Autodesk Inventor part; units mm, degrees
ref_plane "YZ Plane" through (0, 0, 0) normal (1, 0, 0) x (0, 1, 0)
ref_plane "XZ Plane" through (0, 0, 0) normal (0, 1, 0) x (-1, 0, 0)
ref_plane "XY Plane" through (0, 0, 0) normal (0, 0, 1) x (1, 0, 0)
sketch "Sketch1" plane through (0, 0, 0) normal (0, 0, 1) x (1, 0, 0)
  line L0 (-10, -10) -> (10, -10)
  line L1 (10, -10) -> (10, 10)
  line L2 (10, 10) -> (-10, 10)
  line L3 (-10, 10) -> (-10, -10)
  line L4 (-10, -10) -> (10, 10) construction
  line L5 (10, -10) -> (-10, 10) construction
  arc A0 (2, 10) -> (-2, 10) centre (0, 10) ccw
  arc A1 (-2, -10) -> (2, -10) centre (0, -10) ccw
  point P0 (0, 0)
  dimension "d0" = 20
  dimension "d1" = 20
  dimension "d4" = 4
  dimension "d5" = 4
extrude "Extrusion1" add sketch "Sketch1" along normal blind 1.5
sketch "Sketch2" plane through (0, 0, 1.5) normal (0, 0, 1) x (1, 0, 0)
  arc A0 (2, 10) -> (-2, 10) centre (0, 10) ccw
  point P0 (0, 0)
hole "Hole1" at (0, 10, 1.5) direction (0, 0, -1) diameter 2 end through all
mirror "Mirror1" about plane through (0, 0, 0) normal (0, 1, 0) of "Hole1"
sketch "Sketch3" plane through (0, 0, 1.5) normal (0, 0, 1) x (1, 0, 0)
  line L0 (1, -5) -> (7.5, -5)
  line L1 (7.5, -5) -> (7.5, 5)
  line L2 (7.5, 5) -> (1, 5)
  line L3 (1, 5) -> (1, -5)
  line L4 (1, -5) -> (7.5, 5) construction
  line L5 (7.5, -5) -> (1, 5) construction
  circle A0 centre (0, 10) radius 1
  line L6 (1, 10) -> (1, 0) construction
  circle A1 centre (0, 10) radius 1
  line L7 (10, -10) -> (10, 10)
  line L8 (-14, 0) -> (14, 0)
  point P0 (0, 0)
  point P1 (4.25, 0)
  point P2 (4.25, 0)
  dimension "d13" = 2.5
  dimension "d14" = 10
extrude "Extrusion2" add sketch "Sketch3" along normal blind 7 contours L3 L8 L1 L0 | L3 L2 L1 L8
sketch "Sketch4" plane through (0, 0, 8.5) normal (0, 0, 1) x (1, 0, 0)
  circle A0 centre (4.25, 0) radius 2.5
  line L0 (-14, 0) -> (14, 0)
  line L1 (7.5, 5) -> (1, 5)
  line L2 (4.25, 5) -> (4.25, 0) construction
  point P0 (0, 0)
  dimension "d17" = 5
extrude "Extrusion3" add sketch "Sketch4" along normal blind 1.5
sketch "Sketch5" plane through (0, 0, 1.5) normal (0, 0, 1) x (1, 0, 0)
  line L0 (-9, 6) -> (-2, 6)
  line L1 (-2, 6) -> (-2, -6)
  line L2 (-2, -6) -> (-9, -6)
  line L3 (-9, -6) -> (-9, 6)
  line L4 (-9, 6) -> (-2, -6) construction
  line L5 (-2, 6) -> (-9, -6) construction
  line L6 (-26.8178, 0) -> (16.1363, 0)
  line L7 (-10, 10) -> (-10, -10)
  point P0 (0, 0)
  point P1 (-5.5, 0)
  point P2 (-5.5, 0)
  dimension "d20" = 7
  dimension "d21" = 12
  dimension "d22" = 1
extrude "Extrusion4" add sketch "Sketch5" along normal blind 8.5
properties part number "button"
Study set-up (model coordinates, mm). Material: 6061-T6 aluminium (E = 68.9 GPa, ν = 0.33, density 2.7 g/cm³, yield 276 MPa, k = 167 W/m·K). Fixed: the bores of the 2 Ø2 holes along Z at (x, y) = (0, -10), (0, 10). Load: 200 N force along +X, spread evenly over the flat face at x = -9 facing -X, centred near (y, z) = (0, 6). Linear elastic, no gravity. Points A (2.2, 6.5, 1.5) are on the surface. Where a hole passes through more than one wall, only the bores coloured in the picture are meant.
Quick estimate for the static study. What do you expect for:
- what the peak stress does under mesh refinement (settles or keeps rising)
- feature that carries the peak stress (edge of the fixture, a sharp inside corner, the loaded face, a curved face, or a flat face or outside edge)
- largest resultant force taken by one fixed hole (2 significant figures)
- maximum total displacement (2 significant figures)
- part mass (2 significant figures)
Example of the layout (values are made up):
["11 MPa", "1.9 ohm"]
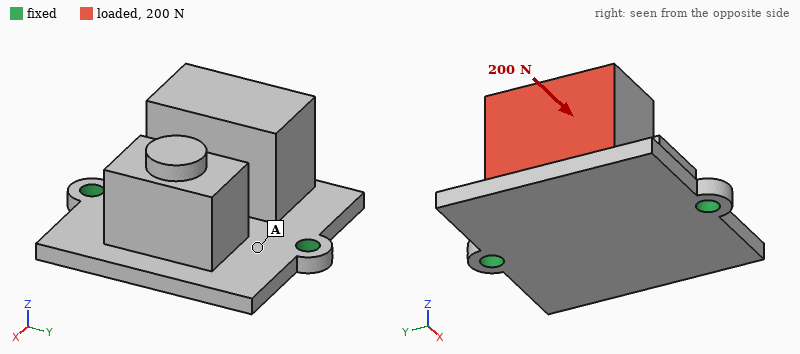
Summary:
["keeps rising", "edge of the fixture", "100 N", "0.14 mm", "4.9 g"]
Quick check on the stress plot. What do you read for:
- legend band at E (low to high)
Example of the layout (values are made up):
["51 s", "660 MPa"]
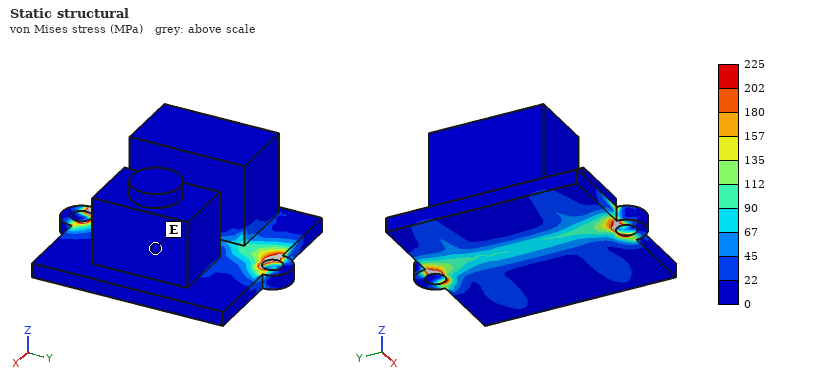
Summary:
["0 to 22 MPa"]
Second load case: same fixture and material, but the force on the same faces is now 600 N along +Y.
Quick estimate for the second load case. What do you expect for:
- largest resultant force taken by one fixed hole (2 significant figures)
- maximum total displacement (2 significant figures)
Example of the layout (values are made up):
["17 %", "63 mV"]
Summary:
["450 N", "40 µm"]
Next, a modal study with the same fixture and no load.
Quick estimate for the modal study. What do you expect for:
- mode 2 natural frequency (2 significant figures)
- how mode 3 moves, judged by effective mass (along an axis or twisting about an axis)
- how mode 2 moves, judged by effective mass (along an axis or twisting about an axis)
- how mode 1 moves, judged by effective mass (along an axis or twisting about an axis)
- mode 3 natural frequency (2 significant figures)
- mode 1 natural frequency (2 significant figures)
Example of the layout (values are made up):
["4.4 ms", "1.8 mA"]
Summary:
["7000 Hz", "along Z", "along Z", "along X", "14 kHz", "3900 Hz"]
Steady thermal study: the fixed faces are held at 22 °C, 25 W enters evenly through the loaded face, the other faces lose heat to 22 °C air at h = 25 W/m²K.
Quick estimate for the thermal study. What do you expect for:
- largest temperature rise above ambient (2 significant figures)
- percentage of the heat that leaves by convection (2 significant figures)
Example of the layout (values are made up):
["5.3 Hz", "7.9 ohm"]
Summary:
["51 K", "4.0 %"]
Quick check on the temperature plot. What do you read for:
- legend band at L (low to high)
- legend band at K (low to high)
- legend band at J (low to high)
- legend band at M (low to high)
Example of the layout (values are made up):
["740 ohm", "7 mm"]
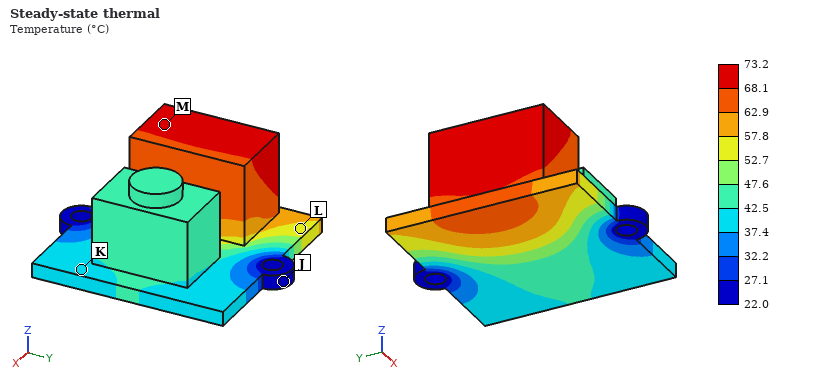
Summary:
["52.7 to 57.8 °C", "37.4 to 42.5 °C", "22.0 to 27.1 °C", "68.1 to 73.2 °C"]
